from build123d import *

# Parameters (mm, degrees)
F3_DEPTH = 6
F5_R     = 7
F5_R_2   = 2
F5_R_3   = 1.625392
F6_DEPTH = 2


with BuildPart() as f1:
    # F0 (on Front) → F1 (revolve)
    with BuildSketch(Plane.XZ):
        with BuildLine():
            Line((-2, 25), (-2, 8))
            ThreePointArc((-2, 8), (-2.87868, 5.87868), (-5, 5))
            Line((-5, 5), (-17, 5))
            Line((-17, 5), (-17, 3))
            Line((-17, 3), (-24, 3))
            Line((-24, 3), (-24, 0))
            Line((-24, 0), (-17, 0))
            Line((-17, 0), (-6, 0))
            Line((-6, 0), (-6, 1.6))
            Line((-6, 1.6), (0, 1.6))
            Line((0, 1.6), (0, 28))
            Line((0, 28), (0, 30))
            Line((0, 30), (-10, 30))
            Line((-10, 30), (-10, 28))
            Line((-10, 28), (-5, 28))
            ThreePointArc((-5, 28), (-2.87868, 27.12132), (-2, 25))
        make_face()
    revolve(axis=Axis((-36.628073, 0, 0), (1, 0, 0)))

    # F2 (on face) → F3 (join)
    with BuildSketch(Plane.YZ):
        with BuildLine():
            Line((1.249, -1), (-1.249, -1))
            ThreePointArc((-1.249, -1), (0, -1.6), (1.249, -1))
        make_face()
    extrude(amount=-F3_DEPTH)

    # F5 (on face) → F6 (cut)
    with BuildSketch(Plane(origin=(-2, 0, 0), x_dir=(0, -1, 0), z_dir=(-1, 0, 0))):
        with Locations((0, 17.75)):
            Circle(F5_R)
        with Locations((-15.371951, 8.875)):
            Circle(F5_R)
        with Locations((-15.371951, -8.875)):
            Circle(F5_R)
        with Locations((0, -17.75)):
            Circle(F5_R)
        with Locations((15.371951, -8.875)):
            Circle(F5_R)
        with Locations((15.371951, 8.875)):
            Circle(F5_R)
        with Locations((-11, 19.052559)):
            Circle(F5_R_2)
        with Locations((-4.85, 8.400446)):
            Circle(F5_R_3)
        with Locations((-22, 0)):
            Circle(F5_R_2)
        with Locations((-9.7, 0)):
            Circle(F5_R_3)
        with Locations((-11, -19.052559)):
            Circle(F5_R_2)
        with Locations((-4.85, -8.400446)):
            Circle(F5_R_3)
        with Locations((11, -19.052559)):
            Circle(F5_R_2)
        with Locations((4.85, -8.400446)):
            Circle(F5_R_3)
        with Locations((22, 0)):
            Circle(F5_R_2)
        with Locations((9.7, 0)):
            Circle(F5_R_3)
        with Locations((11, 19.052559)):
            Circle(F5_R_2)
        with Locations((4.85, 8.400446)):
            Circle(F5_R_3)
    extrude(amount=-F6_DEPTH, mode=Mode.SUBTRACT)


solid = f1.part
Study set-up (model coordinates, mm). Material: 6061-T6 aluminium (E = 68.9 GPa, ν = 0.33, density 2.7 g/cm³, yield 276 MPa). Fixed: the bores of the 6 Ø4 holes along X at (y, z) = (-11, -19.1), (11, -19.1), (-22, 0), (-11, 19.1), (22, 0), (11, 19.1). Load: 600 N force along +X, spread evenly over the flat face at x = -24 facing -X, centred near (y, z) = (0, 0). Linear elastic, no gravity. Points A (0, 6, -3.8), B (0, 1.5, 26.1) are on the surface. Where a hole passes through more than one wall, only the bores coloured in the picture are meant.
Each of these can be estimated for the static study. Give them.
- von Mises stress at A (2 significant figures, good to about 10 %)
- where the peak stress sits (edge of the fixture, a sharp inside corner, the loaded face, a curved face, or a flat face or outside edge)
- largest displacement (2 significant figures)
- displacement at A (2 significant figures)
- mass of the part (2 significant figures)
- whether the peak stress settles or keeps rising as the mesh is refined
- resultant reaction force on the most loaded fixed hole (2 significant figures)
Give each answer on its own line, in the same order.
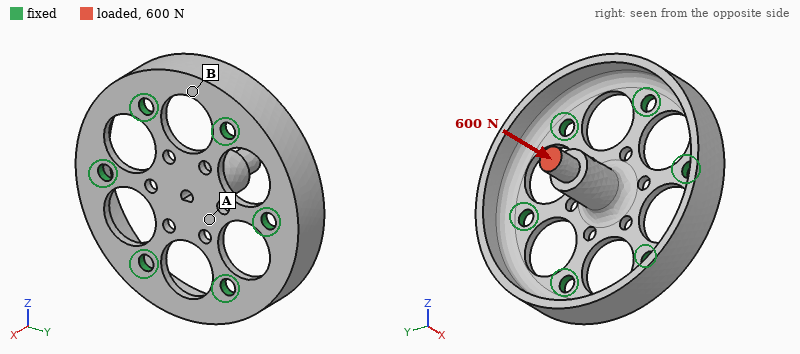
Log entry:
77 MPa
edge of the fixture
0.10 mm
0.097 mm
22 g
keeps rising
100 N
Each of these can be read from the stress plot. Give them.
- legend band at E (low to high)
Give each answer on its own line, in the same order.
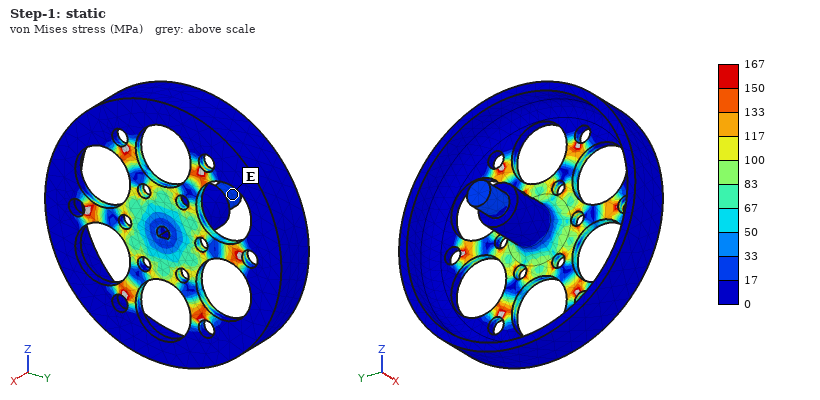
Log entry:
17 to 33 MPa
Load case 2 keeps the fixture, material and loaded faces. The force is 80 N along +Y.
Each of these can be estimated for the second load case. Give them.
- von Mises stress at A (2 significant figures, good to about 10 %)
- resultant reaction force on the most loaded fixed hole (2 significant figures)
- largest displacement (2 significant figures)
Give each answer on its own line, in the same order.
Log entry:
30 MPa
47 N
80 µm
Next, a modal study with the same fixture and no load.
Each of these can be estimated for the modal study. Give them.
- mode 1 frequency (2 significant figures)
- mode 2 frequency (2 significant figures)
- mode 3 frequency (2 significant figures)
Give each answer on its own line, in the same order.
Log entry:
5100 Hz
5100 Hz
5200 Hz
